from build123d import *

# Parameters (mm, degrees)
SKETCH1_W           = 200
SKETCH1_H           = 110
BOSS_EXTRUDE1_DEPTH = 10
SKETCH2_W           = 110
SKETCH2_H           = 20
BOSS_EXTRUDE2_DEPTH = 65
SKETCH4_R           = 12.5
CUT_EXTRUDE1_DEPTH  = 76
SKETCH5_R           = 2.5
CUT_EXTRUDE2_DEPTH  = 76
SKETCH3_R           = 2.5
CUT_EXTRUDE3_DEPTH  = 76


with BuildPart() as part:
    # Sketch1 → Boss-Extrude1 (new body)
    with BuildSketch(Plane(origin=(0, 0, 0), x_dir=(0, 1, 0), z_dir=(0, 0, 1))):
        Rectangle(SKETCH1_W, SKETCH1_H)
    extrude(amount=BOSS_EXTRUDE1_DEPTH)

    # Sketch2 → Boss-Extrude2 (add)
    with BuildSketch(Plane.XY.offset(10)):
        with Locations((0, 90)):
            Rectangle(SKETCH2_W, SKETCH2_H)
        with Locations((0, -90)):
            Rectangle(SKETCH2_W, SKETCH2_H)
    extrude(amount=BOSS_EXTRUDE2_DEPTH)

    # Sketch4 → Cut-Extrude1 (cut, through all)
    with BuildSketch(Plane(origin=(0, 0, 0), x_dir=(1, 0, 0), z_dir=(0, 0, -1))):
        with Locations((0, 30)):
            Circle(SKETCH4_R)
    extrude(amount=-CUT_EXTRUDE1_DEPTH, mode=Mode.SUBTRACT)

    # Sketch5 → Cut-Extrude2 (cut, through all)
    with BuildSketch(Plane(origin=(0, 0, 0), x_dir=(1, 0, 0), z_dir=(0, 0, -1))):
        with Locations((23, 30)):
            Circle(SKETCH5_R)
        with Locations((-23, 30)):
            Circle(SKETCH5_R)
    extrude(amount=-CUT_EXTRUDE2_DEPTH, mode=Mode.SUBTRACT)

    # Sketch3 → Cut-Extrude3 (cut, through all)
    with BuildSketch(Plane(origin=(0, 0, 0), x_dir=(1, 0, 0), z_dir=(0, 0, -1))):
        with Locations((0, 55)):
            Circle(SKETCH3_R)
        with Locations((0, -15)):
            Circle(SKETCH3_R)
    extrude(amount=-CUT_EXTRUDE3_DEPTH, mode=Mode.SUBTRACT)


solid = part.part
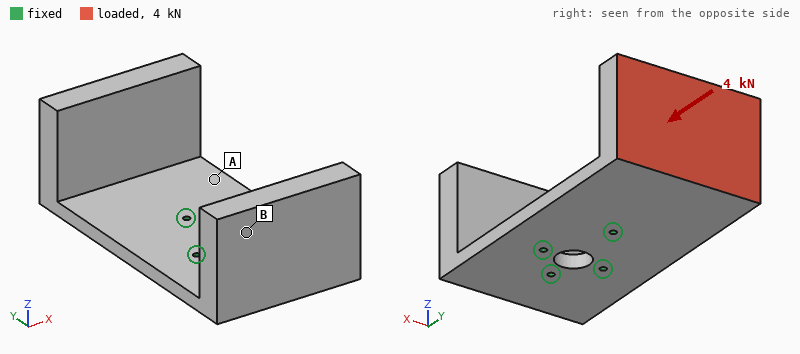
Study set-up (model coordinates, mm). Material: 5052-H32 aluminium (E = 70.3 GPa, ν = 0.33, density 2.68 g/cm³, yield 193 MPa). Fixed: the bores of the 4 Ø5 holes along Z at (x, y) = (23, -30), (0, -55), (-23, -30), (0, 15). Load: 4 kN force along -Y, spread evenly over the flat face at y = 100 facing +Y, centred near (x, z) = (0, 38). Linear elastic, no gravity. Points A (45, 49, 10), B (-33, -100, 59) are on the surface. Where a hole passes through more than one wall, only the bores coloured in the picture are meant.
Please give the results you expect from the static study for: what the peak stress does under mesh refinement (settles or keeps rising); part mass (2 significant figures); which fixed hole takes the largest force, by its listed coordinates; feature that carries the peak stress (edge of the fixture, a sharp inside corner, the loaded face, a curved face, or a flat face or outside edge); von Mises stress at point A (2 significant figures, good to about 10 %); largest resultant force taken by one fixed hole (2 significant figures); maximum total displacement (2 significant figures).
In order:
keeps rising
1.3 kg
(0, 15)
edge of the fixture
70 MPa
3.0 kN
1.3 mm
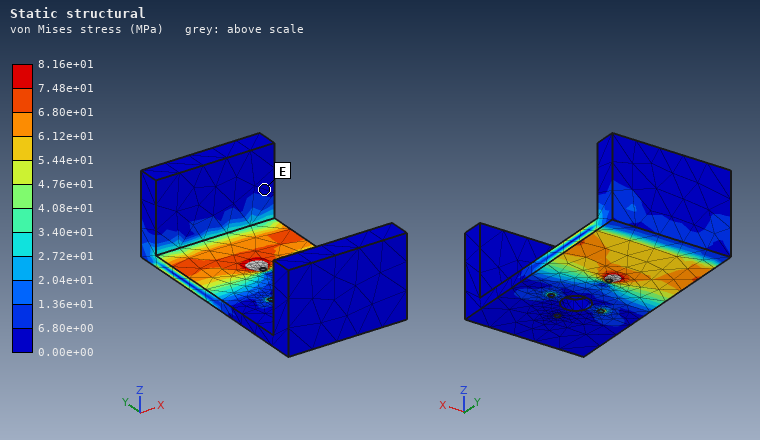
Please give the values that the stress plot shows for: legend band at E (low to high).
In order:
0.00e+00 to 6.80e+00 MPa
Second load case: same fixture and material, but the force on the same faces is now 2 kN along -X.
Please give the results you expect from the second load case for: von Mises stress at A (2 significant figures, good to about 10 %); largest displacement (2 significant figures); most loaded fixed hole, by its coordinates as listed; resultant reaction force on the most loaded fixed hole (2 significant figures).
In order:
23 MPa
0.40 mm
(0, 15)
3.3 kN
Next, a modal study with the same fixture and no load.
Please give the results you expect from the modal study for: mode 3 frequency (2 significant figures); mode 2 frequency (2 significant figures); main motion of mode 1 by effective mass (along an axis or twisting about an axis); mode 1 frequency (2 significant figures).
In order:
680 Hz
550 Hz
along Z
350 Hz
